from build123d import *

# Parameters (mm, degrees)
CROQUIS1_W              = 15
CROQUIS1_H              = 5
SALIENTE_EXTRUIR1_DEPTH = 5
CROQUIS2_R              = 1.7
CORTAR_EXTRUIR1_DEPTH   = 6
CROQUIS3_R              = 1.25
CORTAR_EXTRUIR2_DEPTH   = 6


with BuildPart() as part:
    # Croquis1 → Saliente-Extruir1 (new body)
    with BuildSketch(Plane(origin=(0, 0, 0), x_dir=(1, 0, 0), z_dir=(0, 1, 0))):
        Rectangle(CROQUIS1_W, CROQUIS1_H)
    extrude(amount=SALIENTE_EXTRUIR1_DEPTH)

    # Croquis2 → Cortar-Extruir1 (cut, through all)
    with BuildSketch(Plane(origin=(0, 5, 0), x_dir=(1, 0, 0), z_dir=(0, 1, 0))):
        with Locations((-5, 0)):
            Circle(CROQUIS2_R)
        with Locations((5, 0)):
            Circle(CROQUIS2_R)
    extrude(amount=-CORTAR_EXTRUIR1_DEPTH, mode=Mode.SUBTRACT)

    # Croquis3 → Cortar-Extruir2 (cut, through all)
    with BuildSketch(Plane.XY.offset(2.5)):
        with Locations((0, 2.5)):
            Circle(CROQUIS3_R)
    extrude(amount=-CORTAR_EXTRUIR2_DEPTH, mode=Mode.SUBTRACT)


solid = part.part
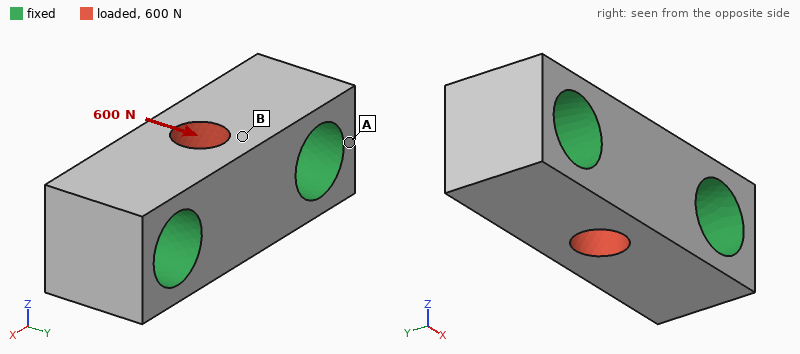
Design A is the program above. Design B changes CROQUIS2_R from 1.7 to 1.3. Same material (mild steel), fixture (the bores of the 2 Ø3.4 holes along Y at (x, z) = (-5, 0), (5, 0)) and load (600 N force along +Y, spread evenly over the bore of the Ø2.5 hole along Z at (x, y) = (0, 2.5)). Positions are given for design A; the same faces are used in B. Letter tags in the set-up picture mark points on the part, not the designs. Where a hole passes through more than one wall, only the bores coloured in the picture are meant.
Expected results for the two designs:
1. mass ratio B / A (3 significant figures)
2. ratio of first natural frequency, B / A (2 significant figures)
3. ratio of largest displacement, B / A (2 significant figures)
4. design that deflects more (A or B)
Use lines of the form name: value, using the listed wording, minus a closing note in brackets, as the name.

mass ratio B / A: 1.15
ratio of first natural frequency, B / A: 0.83
ratio of largest displacement, B / A: 1.2
design that deflects more: B
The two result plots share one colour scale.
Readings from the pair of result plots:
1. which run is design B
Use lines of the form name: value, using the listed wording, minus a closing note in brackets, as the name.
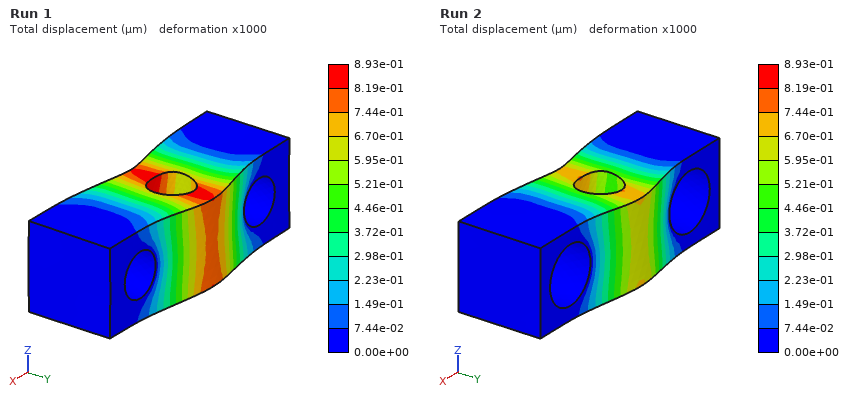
which run is design B: Run 1
